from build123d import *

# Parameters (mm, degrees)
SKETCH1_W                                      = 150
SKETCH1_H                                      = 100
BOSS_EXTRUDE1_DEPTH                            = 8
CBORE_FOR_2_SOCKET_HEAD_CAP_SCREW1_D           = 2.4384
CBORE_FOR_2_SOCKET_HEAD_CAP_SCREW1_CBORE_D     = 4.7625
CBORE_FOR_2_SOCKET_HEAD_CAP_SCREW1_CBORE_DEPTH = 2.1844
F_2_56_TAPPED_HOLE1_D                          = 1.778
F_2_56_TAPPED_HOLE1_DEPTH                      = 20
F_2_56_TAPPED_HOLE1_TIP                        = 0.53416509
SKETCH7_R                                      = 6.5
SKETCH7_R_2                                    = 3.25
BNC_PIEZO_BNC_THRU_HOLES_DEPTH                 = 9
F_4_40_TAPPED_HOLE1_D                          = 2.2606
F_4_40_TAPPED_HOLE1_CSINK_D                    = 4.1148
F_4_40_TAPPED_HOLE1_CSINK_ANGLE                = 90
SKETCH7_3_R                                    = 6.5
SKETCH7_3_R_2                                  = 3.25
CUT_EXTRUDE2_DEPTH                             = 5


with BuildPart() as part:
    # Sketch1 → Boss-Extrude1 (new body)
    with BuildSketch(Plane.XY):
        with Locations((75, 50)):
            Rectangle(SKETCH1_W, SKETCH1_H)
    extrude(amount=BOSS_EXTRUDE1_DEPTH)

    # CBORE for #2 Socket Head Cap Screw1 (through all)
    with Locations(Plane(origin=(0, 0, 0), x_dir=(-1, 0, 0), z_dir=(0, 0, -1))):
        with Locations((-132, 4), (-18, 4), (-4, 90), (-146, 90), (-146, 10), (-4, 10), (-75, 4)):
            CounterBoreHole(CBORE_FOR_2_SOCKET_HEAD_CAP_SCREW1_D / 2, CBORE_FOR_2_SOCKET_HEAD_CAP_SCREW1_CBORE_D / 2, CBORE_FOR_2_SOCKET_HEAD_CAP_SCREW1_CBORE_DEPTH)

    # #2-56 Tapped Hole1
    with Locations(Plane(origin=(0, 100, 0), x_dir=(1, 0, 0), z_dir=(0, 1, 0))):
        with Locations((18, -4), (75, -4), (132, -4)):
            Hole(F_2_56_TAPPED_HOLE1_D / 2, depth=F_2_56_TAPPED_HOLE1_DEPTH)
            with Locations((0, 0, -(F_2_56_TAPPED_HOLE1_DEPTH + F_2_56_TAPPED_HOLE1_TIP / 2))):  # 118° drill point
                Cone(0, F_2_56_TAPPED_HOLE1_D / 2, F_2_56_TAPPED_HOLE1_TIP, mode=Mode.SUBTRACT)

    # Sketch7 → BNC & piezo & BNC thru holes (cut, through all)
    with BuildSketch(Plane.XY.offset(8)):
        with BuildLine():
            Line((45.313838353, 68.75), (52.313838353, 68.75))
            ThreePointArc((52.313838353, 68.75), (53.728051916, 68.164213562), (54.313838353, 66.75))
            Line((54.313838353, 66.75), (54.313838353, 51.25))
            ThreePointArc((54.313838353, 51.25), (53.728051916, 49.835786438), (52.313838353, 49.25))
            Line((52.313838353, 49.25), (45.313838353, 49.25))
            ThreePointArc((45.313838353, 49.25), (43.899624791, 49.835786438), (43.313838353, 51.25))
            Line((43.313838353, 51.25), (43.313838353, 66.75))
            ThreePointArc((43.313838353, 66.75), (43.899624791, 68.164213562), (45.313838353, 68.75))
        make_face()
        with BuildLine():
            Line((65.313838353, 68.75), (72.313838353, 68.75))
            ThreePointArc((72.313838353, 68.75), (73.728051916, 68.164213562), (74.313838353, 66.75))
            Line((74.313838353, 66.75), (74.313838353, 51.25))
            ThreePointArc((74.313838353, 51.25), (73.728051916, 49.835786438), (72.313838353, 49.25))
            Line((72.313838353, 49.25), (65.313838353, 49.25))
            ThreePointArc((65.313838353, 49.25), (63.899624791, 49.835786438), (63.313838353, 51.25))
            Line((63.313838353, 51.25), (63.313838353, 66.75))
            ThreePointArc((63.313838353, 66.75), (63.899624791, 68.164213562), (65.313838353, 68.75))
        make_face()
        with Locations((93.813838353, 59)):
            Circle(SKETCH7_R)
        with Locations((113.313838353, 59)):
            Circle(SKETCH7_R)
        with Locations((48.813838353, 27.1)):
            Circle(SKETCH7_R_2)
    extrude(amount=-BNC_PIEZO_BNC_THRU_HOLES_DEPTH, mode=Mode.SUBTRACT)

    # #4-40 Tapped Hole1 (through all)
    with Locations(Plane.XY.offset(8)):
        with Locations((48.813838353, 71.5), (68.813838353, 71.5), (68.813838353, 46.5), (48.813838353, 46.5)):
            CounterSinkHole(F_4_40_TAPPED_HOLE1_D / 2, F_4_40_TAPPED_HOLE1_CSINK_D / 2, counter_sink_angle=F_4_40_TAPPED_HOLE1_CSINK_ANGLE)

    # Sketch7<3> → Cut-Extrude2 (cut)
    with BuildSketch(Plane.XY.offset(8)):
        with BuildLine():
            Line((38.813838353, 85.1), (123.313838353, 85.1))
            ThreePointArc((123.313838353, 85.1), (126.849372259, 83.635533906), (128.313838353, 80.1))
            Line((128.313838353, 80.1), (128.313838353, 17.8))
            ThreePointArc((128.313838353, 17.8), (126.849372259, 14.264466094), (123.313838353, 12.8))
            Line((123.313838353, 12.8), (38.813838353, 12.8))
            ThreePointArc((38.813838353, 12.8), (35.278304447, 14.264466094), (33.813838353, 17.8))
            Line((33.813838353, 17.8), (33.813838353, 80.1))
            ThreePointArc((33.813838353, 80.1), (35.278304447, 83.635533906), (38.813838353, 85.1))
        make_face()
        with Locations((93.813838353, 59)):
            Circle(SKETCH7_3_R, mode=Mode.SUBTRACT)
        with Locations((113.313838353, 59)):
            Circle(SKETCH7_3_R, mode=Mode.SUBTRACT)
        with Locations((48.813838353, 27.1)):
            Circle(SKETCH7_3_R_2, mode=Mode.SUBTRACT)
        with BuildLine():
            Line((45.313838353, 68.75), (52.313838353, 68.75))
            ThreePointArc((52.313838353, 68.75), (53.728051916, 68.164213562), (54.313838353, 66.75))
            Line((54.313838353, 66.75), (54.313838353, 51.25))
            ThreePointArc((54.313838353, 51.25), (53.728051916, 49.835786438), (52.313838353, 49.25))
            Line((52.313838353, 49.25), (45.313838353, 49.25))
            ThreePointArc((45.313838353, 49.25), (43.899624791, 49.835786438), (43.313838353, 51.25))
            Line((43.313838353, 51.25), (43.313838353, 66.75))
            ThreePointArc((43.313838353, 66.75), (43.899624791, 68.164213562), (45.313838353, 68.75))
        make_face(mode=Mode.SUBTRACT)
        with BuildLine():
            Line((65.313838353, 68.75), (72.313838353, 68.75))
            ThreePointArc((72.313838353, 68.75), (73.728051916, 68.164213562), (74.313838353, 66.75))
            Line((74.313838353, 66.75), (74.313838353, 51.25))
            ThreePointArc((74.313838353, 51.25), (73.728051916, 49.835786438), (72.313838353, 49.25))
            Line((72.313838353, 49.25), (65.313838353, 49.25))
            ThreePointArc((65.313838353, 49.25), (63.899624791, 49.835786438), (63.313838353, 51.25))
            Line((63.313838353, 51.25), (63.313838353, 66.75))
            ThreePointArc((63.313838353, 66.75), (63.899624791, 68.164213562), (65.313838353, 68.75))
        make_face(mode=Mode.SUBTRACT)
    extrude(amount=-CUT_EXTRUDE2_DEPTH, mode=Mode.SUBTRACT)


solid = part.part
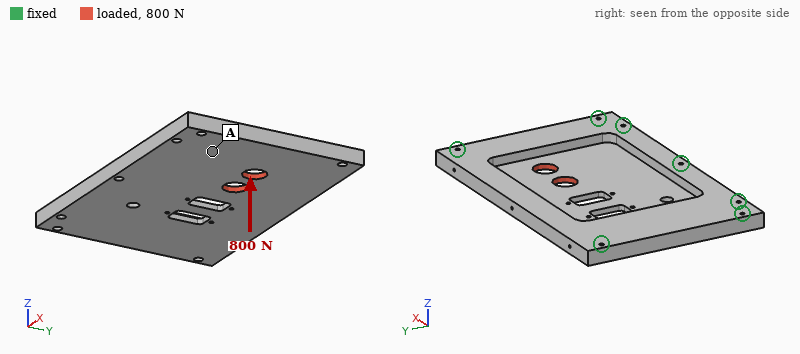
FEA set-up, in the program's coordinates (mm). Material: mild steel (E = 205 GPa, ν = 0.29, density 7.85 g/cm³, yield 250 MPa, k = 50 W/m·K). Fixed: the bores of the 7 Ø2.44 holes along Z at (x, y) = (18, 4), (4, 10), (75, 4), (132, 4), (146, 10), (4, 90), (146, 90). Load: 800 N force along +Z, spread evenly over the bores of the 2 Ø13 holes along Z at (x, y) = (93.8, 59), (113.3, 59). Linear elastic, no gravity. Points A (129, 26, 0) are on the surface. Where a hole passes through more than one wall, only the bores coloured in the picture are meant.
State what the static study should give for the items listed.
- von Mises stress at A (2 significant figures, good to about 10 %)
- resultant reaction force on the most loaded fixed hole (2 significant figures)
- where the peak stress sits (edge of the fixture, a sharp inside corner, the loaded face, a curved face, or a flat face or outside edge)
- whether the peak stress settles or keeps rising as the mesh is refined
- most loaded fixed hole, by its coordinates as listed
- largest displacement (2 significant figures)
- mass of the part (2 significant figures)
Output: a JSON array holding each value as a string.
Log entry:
["13 MPa", "760 N", "edge of the fixture", "keeps rising", "(146, 90)", "77 µm", "650 g"]
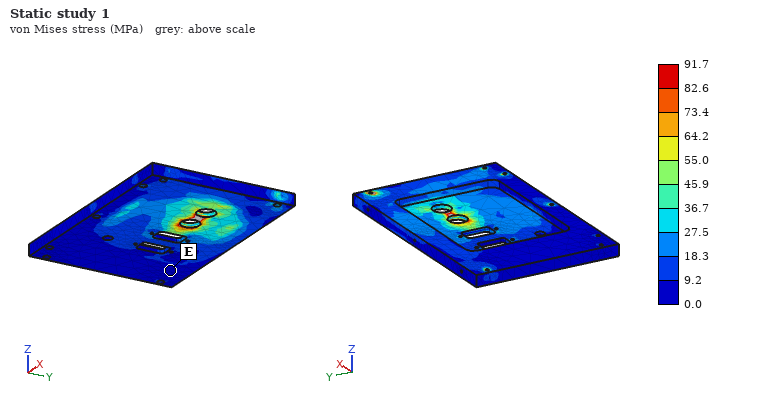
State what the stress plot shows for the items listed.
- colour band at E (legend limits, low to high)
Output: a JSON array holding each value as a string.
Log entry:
["0.0 to 9.2 MPa"]
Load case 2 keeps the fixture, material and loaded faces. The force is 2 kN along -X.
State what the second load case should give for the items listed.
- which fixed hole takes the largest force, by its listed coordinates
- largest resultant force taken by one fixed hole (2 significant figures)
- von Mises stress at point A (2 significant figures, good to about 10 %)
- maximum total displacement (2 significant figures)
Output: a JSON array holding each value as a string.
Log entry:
["(146, 90)", "690 N", "6.4 MPa", "4.8 µm"]
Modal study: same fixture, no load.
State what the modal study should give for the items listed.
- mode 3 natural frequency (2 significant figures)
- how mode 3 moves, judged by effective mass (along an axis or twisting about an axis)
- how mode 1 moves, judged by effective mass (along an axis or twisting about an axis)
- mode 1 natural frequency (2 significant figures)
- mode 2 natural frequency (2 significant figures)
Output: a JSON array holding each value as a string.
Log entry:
["3500 Hz", "twisting about Y", "along Z", "1800 Hz", "3100 Hz"]
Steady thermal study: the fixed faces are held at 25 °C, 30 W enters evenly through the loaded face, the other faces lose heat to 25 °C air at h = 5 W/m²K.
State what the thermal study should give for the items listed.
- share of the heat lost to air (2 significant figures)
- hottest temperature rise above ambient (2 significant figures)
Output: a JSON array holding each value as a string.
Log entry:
["9.7 %", "77 K"]
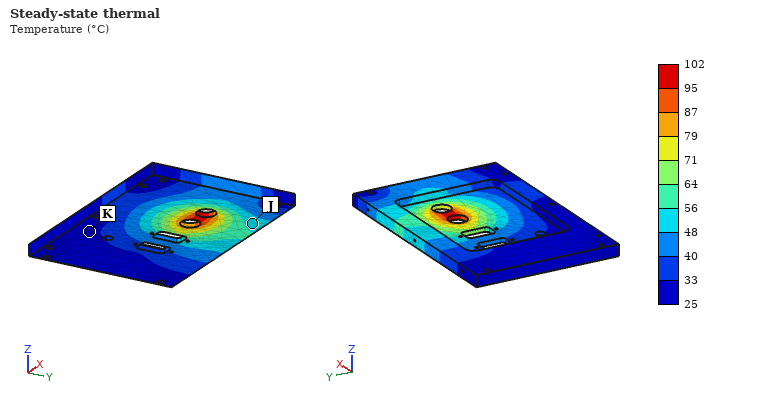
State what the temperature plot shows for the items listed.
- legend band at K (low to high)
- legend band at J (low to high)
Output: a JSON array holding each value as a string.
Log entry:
["25 to 33 °C", "48 to 56 °C"]
